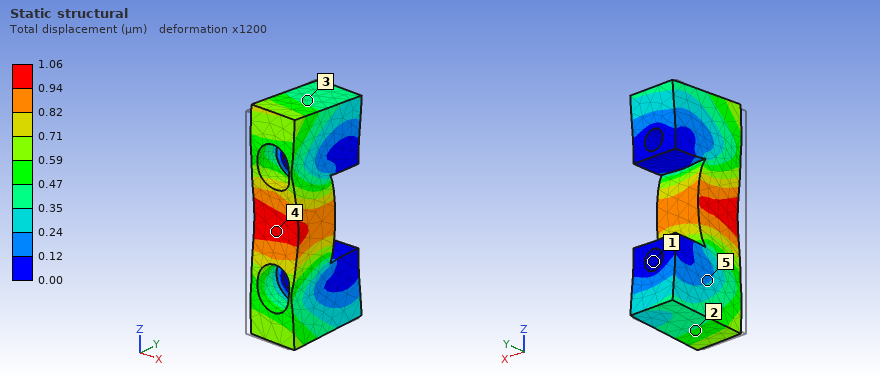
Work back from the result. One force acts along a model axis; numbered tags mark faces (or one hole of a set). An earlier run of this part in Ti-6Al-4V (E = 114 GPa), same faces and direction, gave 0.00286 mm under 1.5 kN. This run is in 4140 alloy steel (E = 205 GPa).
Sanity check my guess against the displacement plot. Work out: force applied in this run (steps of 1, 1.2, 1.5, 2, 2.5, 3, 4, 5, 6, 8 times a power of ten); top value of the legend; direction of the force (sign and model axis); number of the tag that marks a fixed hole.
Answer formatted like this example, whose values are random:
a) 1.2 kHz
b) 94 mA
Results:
a) 1 kN
b) 1.06 µm
c) +Y
d) 1
